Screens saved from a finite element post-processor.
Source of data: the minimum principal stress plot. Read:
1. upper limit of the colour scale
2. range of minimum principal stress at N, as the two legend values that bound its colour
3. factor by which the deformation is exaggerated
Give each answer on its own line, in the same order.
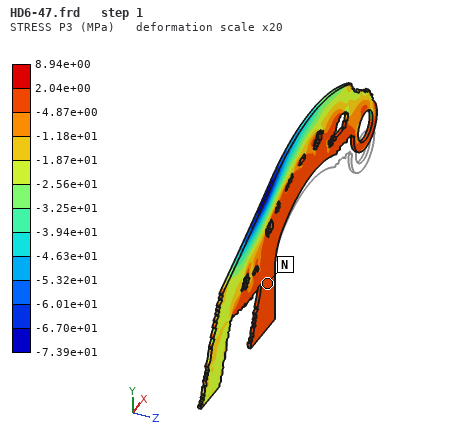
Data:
8.94e+00 MPa
-4.87e+00 to 2.04e+00 MPa
20
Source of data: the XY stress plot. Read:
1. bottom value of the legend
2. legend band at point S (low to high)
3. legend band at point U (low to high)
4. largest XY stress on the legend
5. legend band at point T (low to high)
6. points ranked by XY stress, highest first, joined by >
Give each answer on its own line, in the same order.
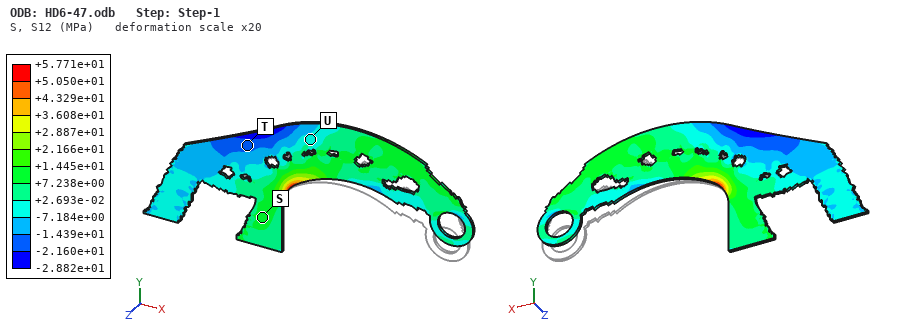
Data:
-2.882e+01 MPa
+7.238e+00 to +1.445e+01 MPa
-7.184e+00 to +2.693e-02 MPa
+5.771e+01 MPa
-2.160e+01 to -1.439e+01 MPa
S > U > T
